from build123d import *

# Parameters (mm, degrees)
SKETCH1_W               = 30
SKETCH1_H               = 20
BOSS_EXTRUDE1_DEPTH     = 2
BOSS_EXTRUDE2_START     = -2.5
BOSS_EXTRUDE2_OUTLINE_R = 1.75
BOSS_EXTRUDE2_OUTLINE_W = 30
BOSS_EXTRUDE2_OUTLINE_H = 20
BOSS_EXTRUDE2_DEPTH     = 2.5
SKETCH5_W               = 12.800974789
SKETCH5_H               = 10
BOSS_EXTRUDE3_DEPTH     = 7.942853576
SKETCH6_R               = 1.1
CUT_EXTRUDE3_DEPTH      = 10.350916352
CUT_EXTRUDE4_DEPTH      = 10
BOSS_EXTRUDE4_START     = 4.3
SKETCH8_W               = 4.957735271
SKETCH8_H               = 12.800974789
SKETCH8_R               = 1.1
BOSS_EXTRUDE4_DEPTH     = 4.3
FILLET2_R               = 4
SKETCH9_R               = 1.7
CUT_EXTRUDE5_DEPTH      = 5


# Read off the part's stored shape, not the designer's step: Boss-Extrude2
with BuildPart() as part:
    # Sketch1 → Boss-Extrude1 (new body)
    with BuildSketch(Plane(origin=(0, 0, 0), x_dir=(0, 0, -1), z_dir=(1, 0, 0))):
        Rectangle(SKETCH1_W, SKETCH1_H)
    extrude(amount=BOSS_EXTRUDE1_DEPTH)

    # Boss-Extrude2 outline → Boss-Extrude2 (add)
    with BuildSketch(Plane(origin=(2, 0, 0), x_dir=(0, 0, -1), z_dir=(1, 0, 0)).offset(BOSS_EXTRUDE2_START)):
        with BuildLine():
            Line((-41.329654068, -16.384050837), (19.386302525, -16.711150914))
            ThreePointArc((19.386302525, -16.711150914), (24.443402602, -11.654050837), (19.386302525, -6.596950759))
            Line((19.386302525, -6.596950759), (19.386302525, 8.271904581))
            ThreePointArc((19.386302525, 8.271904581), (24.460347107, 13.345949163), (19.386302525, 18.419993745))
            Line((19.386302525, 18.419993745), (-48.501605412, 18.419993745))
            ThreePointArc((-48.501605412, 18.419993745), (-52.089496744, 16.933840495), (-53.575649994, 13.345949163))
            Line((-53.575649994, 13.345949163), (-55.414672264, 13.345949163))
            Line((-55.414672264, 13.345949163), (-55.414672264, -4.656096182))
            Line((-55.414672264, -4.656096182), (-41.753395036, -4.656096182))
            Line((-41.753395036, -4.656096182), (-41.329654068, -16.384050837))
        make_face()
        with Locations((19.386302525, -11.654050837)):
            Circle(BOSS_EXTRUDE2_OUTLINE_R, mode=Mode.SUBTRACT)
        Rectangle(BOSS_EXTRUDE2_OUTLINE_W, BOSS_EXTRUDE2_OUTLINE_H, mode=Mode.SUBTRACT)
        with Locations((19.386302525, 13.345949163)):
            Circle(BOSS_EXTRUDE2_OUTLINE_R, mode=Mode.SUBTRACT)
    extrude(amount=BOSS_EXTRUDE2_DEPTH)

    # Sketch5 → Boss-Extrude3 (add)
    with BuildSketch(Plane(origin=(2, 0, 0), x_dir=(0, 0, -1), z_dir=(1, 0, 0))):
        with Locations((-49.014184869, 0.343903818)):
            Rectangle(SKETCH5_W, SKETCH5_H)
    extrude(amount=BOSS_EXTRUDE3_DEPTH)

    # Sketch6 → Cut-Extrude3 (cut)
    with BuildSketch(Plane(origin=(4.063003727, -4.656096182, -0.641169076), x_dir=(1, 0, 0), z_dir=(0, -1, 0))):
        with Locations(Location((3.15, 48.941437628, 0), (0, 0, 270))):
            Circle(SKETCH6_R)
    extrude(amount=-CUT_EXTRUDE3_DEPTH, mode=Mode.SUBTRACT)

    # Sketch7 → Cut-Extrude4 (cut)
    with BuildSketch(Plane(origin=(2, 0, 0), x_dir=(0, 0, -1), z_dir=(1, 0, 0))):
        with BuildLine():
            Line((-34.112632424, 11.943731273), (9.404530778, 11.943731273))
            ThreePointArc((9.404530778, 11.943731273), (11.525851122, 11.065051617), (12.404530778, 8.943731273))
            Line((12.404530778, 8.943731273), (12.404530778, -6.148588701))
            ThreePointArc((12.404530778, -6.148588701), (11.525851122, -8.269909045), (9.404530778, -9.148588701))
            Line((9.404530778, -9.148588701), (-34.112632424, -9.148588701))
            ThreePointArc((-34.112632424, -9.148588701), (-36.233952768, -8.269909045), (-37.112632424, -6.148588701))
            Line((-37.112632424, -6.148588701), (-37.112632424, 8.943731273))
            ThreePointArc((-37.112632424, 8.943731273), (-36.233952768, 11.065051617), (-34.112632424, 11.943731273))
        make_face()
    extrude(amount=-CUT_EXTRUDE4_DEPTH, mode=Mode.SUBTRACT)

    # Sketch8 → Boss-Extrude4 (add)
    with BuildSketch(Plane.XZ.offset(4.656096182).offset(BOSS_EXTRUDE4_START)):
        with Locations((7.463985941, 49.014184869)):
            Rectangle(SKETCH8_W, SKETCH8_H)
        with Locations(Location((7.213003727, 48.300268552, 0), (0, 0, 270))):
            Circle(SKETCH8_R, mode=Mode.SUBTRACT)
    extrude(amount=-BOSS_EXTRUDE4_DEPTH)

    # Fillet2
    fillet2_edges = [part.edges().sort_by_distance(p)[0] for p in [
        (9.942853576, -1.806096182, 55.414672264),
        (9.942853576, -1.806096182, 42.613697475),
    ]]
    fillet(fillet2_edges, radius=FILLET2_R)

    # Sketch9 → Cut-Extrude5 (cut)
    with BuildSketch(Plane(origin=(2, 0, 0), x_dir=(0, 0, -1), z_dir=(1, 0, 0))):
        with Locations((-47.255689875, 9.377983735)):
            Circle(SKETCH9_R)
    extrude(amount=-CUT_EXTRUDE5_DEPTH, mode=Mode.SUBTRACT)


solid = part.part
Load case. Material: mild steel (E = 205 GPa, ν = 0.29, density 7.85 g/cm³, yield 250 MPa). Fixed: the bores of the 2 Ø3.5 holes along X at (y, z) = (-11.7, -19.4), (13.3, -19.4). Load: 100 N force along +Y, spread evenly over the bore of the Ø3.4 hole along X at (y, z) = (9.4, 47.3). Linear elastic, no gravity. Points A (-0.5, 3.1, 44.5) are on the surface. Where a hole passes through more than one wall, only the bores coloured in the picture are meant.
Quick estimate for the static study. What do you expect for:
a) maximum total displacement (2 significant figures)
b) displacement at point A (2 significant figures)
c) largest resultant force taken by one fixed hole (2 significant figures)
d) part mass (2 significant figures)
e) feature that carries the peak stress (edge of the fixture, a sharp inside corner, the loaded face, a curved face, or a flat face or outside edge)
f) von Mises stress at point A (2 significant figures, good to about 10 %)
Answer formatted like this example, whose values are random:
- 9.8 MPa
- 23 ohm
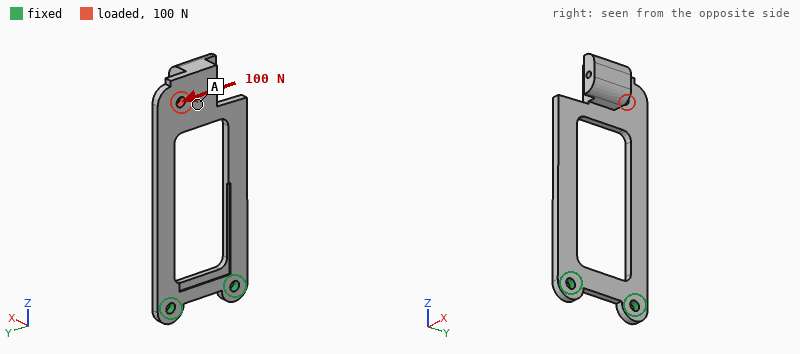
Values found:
- 65 µm
- 63 µm
- 190 N
- 37 g
- a curved face
- 7.9 MPa
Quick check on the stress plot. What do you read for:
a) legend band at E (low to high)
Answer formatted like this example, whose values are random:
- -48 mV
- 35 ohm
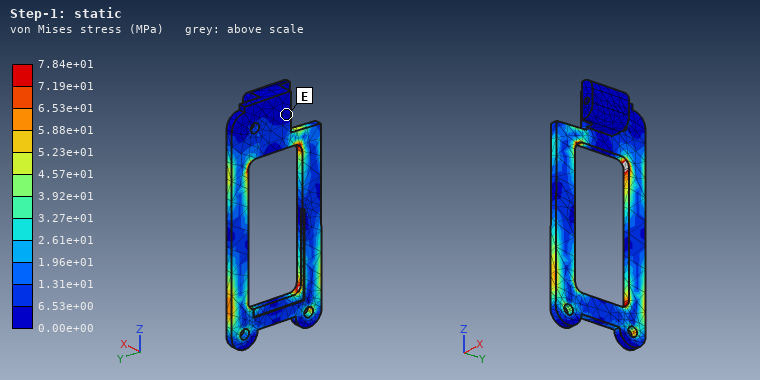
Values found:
- 0.00e+00 to 6.53e+00 MPa
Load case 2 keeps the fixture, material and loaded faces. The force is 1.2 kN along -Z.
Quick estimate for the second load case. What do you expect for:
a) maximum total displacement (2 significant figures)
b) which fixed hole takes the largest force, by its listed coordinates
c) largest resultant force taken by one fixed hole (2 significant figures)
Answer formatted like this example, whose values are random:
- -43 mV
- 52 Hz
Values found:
- 32 µm
- (13.3, -19.4)
- 970 N
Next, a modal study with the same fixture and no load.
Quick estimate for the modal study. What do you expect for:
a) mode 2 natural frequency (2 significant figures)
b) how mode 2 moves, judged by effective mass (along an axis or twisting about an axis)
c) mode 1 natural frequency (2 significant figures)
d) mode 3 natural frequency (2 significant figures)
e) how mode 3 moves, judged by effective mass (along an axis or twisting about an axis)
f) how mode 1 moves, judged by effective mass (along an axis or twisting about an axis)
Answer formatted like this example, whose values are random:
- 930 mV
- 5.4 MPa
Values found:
- 1100 Hz
- along Y
- 230 Hz
- 1400 Hz
- along Y
- along X
